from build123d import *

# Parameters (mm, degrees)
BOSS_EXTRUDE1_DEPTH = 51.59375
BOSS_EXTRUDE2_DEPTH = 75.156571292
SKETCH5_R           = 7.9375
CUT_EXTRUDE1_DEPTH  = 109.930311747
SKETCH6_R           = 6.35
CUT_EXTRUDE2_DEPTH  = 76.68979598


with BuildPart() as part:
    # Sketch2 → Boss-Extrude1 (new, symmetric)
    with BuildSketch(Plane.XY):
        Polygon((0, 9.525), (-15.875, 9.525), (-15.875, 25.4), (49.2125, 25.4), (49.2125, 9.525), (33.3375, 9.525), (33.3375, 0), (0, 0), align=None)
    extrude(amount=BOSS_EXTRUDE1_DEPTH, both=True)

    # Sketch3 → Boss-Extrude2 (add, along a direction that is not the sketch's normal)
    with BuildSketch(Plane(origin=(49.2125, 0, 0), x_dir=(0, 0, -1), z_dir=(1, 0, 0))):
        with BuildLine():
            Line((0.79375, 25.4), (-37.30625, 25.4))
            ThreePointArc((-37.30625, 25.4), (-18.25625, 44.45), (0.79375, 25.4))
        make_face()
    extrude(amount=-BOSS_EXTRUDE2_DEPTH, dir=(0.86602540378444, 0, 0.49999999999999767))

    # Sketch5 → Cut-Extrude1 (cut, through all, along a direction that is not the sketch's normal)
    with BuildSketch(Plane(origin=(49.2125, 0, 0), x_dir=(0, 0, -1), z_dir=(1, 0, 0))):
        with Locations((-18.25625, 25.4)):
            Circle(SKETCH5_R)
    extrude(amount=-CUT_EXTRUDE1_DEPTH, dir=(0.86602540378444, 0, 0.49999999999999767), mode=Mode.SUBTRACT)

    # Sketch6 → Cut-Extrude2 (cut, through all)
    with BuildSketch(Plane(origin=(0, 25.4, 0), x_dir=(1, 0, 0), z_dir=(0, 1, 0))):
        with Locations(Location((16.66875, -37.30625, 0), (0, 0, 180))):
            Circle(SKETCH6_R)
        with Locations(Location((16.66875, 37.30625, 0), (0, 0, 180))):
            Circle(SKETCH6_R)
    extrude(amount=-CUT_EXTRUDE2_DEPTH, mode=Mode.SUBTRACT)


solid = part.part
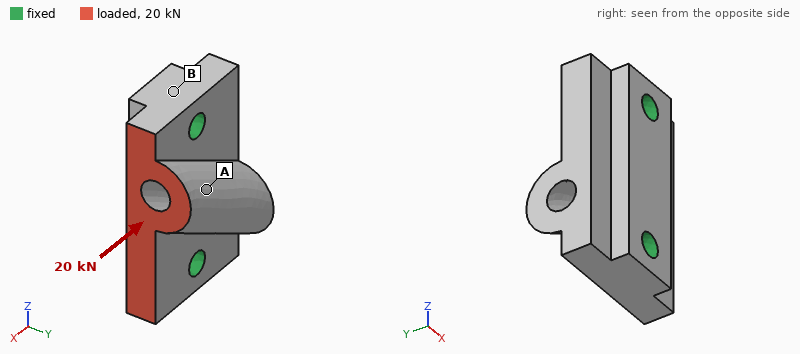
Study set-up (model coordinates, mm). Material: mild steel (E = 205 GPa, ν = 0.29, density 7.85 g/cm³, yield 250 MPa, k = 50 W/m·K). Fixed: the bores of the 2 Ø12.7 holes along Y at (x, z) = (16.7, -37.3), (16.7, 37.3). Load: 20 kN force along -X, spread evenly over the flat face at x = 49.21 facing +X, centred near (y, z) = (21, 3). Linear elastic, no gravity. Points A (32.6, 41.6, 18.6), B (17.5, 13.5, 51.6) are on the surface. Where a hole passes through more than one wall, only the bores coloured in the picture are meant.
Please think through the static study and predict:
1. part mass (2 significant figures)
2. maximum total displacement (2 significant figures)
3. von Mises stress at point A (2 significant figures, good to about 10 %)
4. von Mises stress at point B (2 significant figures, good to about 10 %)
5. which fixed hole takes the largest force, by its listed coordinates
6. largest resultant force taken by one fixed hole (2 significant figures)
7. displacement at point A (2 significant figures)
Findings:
1.2 kg
11 µm
15 MPa
7.1 MPa
(16.7, 37.3)
11 kN
7.3 µm
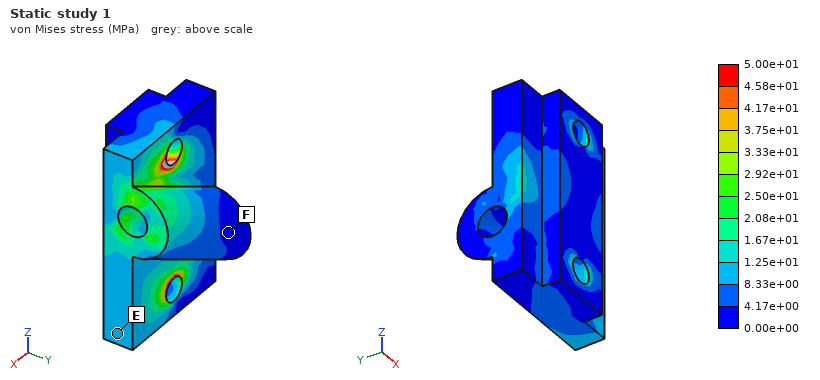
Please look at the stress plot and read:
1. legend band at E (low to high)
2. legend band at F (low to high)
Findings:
8.33e+00 to 1.25e+01 MPa
0.00e+00 to 4.17e+00 MPa
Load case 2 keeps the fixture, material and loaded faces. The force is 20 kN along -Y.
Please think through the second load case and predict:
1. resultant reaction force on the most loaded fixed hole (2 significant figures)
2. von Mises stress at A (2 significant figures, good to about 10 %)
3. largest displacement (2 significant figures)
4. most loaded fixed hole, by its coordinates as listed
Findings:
11 kN
25 MPa
29 µm
(16.7, 37.3)
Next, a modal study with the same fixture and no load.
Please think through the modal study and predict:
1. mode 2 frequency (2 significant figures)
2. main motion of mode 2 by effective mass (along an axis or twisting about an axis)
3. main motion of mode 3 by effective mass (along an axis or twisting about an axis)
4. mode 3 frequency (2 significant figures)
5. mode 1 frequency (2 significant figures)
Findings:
12 kHz
along Y
along X
15 kHz
8700 Hz
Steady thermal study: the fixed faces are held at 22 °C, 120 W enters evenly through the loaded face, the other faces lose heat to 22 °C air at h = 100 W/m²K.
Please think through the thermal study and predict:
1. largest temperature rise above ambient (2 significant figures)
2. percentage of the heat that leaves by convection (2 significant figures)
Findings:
45 K
23 %
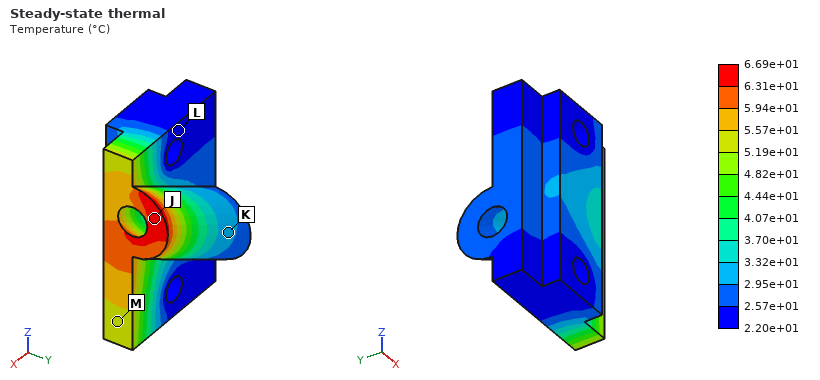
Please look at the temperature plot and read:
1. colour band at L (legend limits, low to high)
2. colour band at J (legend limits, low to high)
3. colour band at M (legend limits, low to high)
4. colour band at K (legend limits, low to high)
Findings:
2.20e+01 to 2.57e+01 °C
6.31e+01 to 6.69e+01 °C
5.19e+01 to 5.57e+01 °C
2.95e+01 to 3.32e+01 °C
